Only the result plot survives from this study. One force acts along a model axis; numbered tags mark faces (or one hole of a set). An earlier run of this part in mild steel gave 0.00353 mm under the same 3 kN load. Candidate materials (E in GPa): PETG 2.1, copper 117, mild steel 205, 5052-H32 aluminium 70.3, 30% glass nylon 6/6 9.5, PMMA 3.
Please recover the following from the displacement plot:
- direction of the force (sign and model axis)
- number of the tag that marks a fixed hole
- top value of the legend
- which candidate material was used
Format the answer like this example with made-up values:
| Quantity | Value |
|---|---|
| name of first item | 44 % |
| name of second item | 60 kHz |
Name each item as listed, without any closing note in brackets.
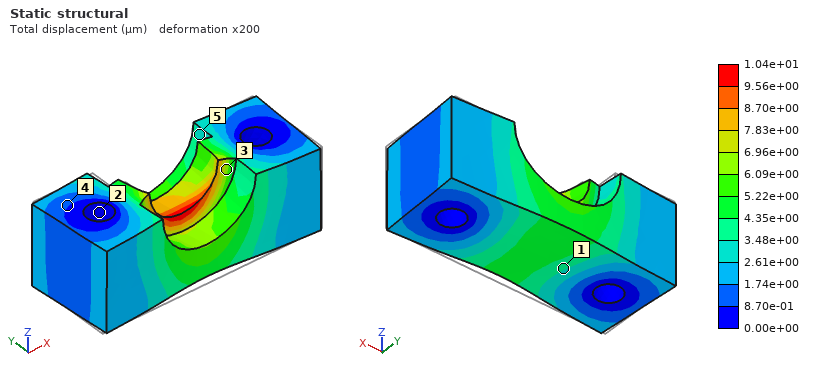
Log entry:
| Quantity | Value |
|---|---|
| direction of the force | +Y |
| number of the tag that marks a fixed hole | 2 |
| top value of the legend | 1.04e+01 µm |
| which candidate material was used | 5052-H32 aluminium |
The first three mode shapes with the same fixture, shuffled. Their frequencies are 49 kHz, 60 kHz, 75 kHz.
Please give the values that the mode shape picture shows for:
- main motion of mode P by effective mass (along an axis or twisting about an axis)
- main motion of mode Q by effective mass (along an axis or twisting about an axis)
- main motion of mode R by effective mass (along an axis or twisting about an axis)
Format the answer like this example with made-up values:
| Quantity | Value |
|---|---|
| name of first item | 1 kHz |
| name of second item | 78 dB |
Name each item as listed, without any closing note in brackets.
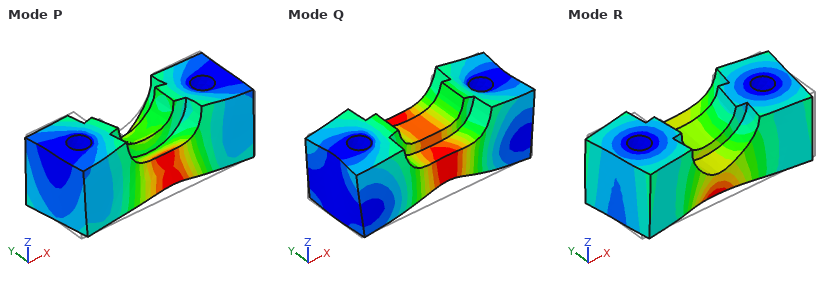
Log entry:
| Quantity | Value |
|---|---|
| main motion of mode P by effective mass | twisting about X |
| main motion of mode Q by effective mass | along Z |
| main motion of mode R by effective mass | along Y |
